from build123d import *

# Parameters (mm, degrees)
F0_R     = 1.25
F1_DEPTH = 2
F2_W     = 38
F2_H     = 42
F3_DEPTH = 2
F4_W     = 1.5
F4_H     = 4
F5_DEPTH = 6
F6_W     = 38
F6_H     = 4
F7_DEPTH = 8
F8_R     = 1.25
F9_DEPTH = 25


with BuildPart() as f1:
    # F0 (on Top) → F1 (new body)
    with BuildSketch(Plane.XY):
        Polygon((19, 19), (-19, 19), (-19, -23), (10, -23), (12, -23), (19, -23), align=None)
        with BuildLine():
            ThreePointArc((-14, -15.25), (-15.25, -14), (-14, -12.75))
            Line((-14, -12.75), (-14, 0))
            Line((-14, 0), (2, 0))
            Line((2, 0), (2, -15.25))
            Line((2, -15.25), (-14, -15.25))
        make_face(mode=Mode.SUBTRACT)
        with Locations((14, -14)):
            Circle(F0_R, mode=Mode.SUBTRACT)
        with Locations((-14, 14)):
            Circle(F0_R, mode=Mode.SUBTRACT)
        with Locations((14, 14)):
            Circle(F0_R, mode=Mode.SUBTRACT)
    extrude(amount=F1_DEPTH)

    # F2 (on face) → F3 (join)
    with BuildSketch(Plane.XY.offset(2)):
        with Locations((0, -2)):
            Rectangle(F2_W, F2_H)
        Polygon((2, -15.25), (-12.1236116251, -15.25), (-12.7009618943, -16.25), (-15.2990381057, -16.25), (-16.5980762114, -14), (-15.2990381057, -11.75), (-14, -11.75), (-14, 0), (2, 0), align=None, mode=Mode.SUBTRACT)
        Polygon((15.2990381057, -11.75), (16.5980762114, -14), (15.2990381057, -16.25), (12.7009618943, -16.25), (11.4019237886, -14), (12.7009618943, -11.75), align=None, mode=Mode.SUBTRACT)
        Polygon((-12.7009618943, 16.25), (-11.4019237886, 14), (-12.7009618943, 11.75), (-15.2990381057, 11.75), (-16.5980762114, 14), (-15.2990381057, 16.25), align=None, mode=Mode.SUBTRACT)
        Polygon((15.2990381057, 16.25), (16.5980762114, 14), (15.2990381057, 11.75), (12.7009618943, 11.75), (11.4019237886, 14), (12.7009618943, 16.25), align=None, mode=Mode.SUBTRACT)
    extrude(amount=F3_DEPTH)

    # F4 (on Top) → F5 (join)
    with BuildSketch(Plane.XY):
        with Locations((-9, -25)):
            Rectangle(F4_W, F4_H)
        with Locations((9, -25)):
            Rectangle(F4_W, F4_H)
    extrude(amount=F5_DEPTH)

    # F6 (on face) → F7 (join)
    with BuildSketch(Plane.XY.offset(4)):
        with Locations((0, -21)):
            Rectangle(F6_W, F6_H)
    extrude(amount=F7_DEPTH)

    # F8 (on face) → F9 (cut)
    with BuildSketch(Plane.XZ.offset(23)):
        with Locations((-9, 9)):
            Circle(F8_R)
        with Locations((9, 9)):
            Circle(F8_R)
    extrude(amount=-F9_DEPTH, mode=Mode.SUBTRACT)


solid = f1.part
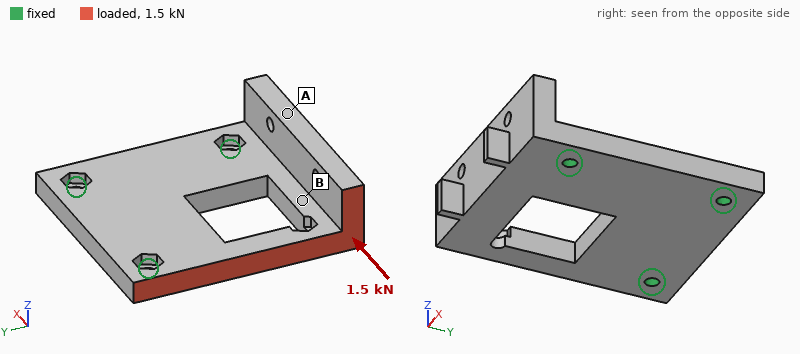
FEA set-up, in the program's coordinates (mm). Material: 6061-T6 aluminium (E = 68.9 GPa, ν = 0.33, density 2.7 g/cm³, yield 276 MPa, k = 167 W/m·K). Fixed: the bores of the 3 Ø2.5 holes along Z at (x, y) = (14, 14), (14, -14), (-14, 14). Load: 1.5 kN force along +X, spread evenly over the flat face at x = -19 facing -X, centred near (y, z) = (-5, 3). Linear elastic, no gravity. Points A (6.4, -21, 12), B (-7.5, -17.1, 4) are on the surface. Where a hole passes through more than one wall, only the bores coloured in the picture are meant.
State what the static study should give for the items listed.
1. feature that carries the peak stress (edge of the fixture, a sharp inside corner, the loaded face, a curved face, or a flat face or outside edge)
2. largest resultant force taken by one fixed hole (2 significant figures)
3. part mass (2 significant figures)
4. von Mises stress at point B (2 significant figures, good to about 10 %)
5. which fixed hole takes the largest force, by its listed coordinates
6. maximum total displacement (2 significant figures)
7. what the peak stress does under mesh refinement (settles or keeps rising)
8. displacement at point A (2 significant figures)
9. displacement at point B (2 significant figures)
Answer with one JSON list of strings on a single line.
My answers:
["edge of the fixture", "770 N", "18 g", "22 MPa", "(14, -14)", "75 µm", "keeps rising", "33 µm", "41 µm"]
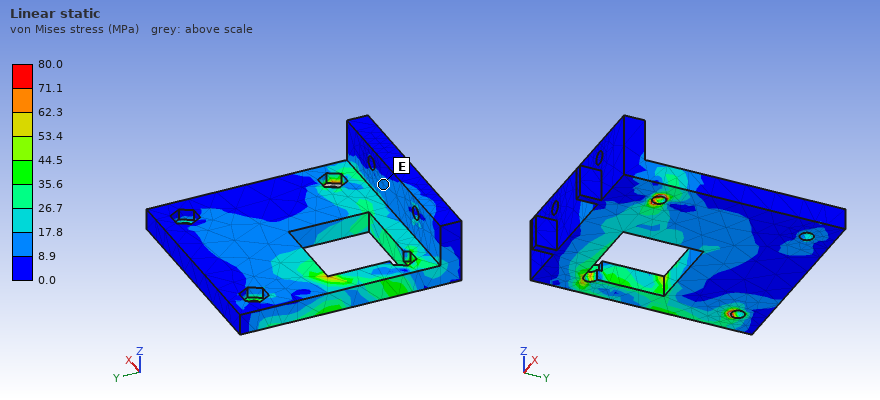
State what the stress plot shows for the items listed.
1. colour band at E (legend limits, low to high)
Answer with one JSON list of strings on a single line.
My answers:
["8.9 to 17.8 MPa"]
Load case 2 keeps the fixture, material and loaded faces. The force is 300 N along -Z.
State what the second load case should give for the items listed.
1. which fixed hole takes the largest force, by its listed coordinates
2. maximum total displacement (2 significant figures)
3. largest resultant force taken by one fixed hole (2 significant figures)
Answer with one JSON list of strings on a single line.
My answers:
["(-14, 14)", "0.20 mm", "300 N"]
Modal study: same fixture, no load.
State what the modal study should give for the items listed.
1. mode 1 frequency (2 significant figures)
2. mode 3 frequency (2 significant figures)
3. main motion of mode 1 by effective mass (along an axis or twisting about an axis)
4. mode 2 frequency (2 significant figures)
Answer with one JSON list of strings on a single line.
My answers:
["3000 Hz", "13 kHz", "along Z", "8200 Hz"]
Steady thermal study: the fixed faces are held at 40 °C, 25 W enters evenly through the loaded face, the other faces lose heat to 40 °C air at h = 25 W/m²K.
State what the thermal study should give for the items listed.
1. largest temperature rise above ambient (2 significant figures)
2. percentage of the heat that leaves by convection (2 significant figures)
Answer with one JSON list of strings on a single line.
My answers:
["34 K", "4.6 %"]
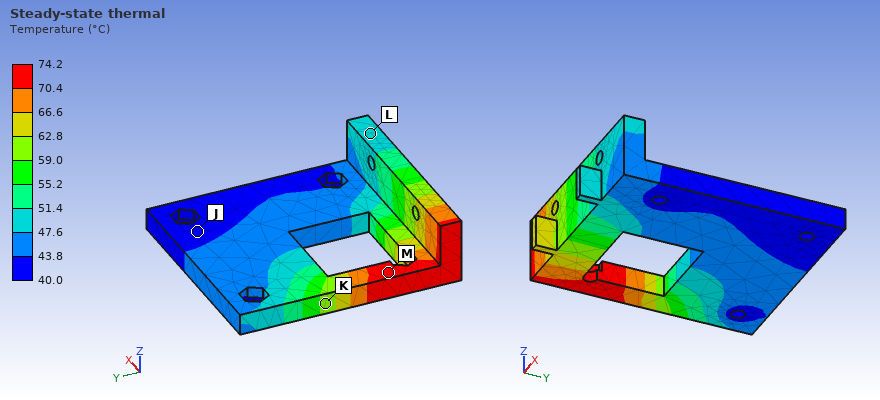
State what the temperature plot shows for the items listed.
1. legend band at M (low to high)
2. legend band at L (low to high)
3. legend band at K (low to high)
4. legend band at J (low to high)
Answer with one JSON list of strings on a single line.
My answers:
["70.4 to 74.2 °C", "47.6 to 51.4 °C", "59.0 to 62.8 °C", "40.0 to 43.8 °C"]
